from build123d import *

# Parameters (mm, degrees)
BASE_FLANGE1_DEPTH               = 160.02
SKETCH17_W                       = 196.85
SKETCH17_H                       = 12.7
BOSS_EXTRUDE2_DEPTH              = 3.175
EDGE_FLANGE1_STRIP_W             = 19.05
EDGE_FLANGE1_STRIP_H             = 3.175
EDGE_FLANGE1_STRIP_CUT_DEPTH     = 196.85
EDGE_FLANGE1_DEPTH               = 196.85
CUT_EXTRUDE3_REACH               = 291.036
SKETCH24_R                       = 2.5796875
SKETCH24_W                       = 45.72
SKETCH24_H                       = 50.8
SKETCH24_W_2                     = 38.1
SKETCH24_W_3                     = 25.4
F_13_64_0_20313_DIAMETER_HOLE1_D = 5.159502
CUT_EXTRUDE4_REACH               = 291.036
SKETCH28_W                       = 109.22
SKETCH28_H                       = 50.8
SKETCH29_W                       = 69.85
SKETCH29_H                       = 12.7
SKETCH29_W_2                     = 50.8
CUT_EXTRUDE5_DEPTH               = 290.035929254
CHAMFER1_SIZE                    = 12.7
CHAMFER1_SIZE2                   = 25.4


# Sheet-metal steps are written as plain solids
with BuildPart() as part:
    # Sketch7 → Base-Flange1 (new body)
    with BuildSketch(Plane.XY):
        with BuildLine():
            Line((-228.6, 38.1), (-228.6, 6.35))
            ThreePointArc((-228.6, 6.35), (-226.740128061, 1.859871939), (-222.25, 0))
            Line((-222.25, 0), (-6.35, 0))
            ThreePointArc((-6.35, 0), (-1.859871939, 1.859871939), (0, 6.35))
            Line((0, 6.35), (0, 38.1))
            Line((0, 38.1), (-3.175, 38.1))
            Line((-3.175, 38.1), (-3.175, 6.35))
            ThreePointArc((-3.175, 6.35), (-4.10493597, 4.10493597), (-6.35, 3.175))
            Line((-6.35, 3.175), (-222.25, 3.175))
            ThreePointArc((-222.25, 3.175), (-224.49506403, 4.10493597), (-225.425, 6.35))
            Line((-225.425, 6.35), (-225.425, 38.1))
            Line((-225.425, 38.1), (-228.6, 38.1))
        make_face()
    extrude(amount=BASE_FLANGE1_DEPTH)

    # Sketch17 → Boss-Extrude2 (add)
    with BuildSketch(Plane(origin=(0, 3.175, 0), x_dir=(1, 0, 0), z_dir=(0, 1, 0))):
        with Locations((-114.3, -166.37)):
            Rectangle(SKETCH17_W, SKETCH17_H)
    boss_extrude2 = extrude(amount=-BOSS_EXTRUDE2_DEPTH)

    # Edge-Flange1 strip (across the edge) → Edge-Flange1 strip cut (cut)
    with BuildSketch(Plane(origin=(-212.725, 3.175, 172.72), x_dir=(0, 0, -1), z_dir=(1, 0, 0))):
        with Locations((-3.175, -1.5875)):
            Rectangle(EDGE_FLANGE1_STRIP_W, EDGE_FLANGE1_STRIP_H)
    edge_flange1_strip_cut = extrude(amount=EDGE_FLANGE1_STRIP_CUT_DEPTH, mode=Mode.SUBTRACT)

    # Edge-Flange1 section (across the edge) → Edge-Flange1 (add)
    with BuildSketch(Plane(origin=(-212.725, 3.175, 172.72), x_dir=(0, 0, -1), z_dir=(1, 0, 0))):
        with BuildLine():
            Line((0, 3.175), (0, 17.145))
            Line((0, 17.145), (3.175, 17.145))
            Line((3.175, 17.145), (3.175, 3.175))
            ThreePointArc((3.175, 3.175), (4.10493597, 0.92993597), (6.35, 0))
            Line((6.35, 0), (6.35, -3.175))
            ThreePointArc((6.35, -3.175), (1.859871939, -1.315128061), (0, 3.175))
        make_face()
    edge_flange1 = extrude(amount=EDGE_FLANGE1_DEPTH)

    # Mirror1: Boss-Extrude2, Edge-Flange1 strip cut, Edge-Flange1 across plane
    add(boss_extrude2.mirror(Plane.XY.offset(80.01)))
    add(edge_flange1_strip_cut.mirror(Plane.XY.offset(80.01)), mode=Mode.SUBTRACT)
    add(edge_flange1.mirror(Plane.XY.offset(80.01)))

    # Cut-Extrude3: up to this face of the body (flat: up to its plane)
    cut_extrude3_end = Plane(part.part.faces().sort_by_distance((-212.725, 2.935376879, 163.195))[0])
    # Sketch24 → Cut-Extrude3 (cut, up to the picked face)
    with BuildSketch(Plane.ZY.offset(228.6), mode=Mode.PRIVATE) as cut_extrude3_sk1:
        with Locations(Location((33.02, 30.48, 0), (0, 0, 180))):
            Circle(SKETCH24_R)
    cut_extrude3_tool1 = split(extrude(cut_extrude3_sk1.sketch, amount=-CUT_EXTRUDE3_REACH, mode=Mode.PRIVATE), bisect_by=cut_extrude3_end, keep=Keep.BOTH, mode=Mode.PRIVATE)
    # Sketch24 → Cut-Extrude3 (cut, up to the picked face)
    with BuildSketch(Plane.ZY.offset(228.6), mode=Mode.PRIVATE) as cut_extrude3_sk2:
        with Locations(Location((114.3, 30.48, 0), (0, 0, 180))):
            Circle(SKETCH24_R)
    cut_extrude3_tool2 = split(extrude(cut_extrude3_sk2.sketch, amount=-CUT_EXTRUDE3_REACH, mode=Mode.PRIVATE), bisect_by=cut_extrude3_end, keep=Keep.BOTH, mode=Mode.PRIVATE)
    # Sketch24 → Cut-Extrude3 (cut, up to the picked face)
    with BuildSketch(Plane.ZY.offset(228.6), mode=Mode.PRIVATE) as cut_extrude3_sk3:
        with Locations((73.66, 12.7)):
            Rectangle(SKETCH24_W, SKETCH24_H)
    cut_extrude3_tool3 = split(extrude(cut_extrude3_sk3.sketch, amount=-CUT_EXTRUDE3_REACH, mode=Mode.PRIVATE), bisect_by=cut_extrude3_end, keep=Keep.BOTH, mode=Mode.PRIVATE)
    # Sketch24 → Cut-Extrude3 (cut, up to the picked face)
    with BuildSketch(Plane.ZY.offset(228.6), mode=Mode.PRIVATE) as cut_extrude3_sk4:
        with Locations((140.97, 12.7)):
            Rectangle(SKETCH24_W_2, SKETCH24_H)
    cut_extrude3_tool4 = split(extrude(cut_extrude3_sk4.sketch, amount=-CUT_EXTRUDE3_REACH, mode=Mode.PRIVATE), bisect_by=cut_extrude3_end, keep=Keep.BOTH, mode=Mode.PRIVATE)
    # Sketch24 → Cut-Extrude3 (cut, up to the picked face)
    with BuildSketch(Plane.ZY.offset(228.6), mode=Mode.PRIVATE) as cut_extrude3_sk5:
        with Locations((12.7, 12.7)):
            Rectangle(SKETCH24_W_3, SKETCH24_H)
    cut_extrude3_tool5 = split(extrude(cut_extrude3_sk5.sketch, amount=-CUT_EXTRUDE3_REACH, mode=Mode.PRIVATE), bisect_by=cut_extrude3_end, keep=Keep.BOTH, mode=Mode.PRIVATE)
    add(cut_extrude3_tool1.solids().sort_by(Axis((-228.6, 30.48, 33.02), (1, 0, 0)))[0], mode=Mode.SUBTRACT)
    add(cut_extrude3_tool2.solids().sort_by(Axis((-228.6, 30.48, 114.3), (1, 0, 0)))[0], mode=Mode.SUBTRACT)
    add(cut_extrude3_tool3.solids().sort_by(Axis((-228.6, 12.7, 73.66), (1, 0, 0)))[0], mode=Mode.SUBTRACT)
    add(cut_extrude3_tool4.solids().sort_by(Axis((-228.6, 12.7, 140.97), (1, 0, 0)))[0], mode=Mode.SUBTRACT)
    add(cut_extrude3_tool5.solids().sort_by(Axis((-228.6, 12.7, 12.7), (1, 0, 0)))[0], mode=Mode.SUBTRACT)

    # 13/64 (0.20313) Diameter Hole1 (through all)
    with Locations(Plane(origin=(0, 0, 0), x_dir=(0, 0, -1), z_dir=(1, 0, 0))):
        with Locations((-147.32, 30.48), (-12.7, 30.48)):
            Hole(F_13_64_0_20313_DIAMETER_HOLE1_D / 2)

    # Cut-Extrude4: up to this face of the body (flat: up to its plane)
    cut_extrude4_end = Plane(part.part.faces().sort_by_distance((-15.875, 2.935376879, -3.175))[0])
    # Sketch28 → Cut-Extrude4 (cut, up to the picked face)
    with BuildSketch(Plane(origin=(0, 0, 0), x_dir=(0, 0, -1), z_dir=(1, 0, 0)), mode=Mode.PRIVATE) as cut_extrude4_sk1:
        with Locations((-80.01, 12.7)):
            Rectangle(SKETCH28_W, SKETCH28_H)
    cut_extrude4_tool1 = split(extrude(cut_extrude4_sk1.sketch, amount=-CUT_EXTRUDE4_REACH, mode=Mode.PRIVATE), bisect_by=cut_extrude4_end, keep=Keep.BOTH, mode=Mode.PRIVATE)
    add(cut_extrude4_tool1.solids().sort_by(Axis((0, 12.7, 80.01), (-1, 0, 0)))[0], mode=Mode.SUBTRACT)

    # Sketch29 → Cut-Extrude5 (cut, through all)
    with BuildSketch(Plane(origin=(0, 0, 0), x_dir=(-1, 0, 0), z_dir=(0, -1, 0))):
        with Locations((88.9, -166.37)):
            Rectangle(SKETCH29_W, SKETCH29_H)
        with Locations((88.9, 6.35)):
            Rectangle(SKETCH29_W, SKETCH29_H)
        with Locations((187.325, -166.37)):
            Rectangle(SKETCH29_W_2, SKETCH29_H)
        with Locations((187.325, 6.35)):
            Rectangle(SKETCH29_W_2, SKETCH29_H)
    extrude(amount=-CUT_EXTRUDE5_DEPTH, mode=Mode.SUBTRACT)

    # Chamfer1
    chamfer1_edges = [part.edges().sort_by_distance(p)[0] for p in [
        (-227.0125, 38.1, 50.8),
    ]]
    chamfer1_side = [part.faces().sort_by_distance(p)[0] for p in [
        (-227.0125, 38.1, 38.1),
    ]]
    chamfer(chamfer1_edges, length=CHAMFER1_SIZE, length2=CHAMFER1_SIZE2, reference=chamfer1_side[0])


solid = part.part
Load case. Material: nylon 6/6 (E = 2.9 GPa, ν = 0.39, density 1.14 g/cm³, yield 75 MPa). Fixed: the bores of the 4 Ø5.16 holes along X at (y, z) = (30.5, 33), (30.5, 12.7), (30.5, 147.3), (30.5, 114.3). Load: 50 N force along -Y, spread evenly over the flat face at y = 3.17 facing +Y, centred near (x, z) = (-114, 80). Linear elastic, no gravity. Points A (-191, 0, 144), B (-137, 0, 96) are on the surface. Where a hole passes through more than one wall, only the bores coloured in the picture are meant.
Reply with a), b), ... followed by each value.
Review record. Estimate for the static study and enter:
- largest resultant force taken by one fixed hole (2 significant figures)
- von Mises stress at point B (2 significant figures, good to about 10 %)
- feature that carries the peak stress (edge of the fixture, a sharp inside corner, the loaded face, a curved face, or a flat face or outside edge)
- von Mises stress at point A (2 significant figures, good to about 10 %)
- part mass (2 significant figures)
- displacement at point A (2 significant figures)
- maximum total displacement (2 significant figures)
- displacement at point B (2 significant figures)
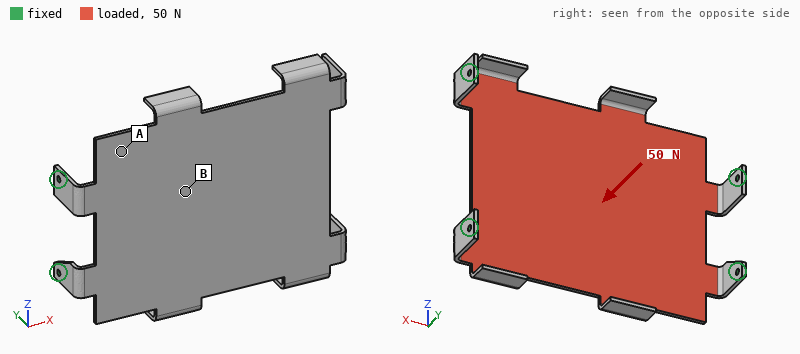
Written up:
a) 24 N
b) 2.4 MPa
c) a curved face
d) 0.96 MPa
e) 150 g
f) 1.3 mm
g) 3.0 mm
h) 2.3 mm
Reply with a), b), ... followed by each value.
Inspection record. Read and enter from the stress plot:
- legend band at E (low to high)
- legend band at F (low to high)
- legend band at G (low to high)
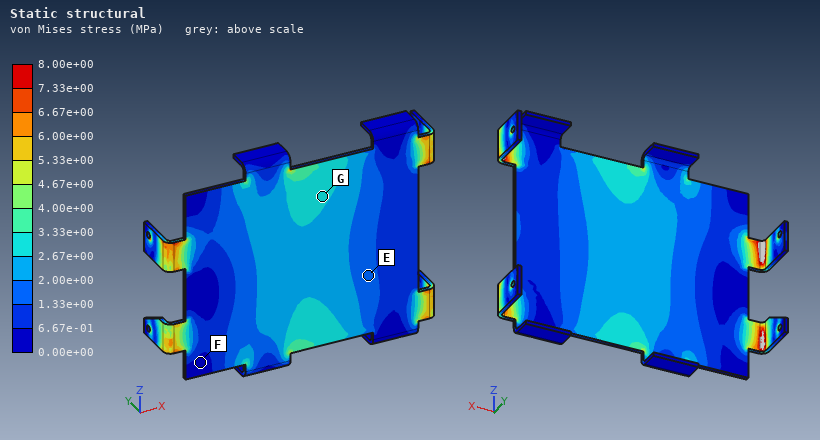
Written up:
a) 1.33e+00 to 2.00e+00 MPa
b) 0.00e+00 to 6.67e-01 MPa
c) 2.67e+00 to 3.33e+00 MPa
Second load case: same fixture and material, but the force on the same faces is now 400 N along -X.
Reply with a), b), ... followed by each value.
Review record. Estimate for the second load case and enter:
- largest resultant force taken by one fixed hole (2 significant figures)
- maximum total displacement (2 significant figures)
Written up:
a) 100 N
b) 3.2 mm
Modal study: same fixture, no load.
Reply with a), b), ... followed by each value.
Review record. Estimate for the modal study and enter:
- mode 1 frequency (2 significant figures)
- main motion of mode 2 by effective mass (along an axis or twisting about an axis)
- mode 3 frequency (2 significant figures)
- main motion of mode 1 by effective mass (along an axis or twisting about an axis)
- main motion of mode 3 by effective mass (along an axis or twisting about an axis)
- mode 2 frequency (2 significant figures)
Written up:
a) 69 Hz
b) twisting about X
c) 150 Hz
d) along Y
e) along X
f) 90 Hz
